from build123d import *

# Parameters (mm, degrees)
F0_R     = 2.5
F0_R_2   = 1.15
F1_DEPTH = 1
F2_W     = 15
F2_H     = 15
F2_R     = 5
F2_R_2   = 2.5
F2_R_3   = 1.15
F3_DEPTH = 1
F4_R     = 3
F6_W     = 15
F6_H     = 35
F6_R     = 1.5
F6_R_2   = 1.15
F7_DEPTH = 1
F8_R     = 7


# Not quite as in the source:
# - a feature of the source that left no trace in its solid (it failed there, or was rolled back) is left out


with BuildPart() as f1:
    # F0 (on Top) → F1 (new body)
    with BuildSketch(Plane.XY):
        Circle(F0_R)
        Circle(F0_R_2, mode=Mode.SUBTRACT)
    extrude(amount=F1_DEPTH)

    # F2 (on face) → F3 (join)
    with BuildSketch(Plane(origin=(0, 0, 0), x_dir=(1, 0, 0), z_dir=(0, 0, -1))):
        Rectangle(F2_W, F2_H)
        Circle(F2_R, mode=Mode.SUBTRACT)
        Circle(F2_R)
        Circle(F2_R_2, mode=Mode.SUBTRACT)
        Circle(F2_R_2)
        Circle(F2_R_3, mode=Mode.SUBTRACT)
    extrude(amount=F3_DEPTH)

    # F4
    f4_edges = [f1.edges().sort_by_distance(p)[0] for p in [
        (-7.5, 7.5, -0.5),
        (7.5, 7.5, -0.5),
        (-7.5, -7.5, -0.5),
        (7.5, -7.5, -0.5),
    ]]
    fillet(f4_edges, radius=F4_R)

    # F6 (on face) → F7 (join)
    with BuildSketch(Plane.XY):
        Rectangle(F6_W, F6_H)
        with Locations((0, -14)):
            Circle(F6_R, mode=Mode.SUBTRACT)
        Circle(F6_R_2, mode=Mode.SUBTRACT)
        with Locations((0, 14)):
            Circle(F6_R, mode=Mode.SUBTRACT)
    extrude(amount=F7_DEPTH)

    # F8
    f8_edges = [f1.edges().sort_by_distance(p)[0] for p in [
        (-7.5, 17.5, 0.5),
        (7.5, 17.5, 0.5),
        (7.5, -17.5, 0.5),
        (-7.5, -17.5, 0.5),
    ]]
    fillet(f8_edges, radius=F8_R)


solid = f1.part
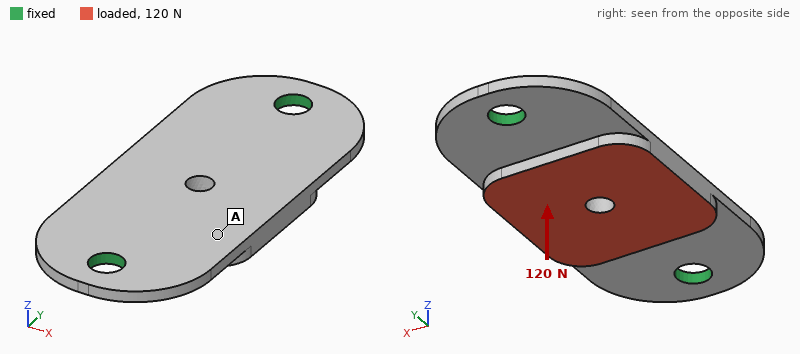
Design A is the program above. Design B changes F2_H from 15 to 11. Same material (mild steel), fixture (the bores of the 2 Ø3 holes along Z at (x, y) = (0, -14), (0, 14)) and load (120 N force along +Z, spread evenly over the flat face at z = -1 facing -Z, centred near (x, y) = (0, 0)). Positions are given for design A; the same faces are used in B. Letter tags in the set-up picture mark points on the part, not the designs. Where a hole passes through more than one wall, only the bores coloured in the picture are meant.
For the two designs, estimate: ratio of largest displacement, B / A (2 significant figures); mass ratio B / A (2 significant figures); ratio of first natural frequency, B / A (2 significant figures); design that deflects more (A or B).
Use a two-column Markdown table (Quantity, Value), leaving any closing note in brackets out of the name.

| Quantity | Value |
|---|---|
| ratio of largest displacement, B / A | 1.4 |
| mass ratio B / A | 0.91 |
| ratio of first natural frequency, B / A | 0.97 |
| design that deflects more | B |
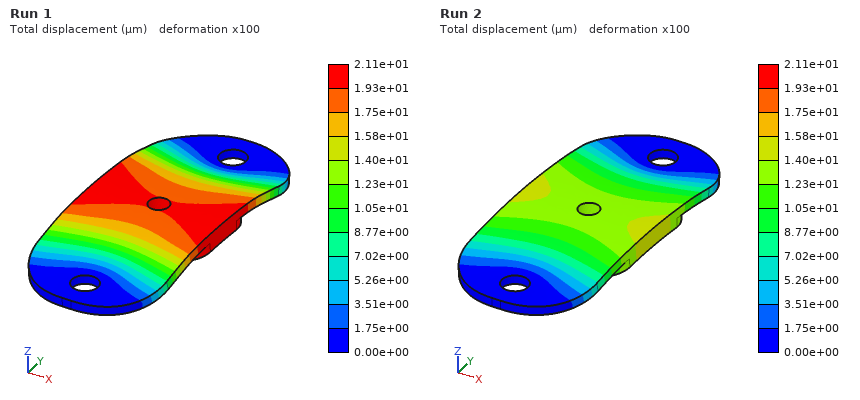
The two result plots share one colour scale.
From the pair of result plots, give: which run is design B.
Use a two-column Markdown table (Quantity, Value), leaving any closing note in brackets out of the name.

| Quantity | Value |
|---|---|
| which run is design B | Run 1 |
